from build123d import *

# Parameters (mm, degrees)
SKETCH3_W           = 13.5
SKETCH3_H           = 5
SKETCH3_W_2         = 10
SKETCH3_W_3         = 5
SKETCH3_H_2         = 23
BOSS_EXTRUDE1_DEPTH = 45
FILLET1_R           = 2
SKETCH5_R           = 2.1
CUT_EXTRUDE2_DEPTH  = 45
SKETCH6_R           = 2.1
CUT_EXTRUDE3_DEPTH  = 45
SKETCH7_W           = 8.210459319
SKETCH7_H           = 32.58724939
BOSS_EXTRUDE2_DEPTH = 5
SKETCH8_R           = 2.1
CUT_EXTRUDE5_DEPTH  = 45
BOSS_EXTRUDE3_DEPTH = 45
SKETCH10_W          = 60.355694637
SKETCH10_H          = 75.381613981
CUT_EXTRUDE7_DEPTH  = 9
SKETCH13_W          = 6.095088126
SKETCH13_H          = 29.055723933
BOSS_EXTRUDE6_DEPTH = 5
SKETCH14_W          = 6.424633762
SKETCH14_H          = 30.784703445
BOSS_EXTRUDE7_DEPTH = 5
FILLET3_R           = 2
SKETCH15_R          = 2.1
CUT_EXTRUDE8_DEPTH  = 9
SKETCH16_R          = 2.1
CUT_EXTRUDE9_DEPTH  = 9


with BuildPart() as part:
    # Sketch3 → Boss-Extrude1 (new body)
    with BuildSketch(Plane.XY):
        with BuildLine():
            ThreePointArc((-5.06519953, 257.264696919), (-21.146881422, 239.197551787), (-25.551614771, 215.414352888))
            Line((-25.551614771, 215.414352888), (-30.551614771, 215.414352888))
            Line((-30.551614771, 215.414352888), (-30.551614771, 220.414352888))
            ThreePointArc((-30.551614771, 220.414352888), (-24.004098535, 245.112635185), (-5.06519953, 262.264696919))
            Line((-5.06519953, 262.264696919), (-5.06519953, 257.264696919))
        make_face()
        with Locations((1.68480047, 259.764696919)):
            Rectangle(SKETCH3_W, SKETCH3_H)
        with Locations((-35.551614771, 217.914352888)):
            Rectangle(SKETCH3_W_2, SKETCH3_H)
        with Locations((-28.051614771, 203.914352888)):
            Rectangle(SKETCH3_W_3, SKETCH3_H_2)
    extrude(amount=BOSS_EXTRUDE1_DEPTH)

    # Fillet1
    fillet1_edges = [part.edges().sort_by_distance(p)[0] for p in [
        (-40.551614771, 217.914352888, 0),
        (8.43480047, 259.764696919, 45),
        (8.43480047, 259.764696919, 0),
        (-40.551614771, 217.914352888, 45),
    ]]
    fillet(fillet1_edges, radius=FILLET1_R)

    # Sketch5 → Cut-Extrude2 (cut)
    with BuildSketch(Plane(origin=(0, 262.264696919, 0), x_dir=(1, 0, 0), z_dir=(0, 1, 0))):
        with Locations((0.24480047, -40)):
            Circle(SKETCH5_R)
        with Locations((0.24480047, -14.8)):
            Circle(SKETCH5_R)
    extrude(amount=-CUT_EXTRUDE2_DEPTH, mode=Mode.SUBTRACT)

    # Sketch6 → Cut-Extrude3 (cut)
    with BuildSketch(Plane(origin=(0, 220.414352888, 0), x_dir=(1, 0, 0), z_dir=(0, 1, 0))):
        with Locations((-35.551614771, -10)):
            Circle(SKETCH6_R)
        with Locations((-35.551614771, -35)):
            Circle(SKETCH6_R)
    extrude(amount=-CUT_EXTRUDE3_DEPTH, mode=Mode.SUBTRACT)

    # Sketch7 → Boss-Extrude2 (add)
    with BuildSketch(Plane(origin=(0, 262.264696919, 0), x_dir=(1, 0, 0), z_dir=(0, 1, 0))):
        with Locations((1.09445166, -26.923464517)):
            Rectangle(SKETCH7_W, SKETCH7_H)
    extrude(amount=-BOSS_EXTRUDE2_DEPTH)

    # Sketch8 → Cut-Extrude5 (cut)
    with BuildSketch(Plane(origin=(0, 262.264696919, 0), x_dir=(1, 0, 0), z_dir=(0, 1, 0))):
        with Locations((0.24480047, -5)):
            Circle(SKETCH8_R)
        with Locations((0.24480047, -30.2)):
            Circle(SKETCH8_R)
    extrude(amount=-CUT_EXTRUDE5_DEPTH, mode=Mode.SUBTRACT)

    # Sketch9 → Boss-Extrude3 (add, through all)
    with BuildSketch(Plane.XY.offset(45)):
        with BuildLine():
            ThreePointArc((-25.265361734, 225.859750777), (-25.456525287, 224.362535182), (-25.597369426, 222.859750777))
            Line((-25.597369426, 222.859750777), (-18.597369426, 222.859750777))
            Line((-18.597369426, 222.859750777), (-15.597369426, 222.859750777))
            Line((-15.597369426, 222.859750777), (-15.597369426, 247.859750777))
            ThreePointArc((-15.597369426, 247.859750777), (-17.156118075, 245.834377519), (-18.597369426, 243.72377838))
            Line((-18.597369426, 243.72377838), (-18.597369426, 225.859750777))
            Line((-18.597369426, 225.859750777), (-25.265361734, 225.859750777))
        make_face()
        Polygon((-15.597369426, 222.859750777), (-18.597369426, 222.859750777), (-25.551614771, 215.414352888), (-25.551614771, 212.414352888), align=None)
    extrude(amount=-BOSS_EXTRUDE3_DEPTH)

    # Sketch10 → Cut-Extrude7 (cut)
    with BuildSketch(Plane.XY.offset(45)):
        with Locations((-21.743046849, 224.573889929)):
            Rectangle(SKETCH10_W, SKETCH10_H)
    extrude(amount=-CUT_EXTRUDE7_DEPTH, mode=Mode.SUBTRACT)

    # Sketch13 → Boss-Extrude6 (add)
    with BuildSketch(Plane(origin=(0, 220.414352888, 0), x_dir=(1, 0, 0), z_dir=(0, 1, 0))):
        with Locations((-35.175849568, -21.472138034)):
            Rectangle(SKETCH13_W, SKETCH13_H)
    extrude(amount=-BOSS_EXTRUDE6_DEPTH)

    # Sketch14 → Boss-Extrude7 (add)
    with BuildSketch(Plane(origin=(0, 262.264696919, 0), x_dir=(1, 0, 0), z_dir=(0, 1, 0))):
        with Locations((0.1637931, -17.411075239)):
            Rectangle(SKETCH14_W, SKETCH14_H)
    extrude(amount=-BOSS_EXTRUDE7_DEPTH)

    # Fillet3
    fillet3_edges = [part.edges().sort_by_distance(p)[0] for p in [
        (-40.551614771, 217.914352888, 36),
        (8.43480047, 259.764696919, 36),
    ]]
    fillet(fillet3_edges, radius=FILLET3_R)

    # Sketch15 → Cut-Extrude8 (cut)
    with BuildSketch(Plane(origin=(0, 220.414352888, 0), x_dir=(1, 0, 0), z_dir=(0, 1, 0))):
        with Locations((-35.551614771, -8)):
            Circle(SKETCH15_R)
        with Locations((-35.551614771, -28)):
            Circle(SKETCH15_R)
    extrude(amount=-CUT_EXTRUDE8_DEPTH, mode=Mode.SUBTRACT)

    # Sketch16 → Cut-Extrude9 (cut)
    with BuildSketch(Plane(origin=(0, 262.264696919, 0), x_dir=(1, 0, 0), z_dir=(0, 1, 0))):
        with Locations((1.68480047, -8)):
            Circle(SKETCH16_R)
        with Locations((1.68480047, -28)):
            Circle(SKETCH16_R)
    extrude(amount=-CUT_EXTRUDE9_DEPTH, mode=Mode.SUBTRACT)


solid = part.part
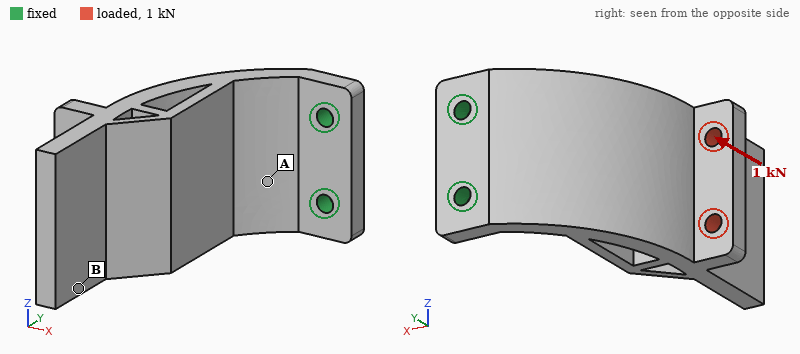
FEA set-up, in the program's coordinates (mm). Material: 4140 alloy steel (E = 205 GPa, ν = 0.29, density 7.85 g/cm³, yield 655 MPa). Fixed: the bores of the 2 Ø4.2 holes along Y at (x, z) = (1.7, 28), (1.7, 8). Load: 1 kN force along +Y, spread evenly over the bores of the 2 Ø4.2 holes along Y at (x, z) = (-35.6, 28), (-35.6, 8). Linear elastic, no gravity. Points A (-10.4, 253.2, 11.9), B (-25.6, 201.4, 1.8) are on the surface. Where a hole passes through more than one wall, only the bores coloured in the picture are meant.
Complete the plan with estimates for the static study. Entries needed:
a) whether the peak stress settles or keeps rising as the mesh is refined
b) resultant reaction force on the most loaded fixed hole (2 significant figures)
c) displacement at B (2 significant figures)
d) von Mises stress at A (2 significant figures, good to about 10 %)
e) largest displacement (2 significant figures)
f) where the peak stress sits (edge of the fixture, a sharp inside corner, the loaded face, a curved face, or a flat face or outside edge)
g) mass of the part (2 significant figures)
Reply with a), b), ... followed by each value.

a) keeps rising
b) 520 N
c) 0.54 mm
d) 160 MPa
e) 0.64 mm
f) edge of the fixture
g) 170 g
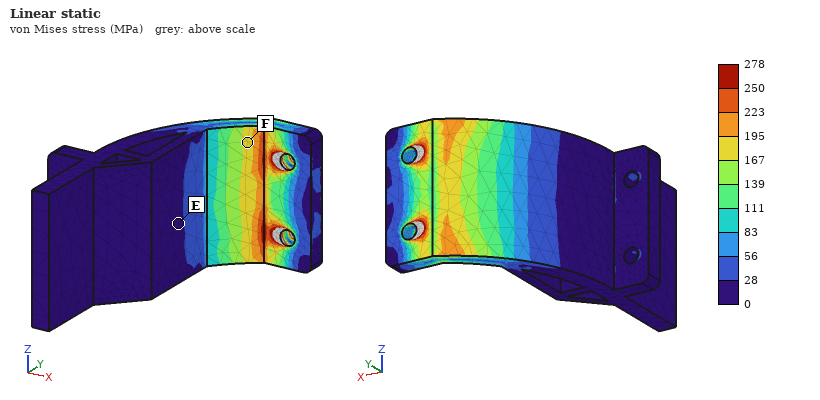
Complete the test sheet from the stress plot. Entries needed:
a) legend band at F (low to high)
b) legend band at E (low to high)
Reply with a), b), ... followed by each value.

a) 167 to 195 MPa
b) 0 to 28 MPa
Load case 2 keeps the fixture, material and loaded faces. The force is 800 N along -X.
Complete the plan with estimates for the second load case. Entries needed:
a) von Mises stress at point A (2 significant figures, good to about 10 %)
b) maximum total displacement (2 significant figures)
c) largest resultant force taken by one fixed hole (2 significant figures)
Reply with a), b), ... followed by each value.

a) 200 MPa
b) 0.74 mm
c) 450 N
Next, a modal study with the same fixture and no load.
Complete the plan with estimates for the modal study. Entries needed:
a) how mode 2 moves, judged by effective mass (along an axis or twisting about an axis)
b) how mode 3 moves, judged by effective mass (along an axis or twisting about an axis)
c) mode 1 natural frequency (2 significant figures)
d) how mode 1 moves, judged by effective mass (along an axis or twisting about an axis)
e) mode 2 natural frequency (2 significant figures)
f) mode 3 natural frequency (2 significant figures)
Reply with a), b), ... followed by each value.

a) along Z
b) along Y
c) 580 Hz
d) along X
e) 1500 Hz
f) 4200 Hz
